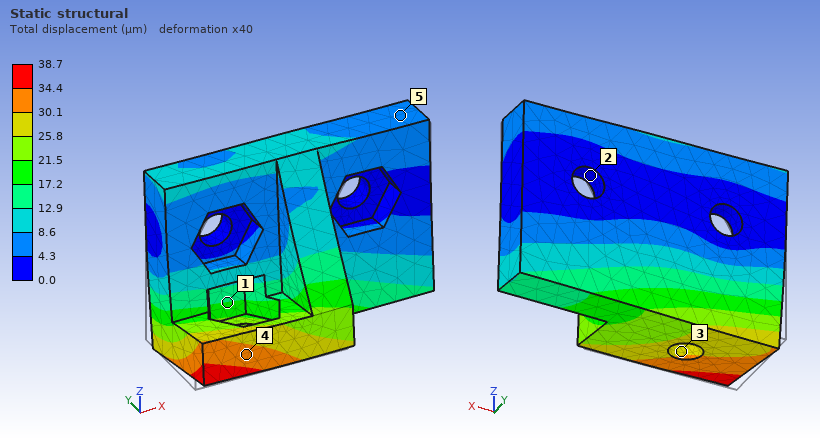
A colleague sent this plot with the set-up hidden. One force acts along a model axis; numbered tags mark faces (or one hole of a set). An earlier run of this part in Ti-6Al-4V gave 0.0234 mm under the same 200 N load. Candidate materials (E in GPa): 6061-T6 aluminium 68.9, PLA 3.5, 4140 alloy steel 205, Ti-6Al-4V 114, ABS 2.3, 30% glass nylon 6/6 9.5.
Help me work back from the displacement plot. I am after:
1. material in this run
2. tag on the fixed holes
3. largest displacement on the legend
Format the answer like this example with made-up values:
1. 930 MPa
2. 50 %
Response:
1. 6061-T6 aluminium
2. 2
3. 38.7 µm
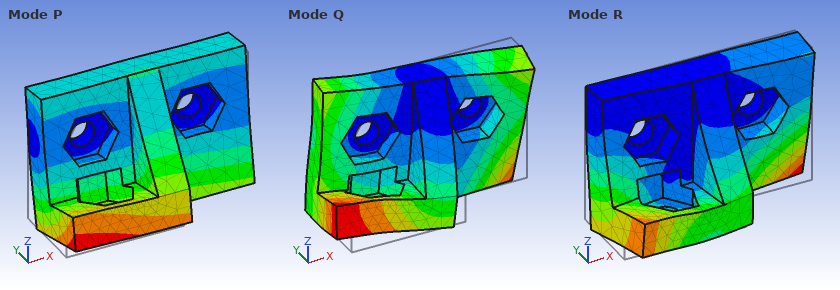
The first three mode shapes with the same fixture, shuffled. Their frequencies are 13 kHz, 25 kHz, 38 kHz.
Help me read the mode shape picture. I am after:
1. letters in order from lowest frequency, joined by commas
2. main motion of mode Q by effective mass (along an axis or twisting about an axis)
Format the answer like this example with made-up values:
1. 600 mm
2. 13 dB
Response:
1. P, R, Q
2. along X
